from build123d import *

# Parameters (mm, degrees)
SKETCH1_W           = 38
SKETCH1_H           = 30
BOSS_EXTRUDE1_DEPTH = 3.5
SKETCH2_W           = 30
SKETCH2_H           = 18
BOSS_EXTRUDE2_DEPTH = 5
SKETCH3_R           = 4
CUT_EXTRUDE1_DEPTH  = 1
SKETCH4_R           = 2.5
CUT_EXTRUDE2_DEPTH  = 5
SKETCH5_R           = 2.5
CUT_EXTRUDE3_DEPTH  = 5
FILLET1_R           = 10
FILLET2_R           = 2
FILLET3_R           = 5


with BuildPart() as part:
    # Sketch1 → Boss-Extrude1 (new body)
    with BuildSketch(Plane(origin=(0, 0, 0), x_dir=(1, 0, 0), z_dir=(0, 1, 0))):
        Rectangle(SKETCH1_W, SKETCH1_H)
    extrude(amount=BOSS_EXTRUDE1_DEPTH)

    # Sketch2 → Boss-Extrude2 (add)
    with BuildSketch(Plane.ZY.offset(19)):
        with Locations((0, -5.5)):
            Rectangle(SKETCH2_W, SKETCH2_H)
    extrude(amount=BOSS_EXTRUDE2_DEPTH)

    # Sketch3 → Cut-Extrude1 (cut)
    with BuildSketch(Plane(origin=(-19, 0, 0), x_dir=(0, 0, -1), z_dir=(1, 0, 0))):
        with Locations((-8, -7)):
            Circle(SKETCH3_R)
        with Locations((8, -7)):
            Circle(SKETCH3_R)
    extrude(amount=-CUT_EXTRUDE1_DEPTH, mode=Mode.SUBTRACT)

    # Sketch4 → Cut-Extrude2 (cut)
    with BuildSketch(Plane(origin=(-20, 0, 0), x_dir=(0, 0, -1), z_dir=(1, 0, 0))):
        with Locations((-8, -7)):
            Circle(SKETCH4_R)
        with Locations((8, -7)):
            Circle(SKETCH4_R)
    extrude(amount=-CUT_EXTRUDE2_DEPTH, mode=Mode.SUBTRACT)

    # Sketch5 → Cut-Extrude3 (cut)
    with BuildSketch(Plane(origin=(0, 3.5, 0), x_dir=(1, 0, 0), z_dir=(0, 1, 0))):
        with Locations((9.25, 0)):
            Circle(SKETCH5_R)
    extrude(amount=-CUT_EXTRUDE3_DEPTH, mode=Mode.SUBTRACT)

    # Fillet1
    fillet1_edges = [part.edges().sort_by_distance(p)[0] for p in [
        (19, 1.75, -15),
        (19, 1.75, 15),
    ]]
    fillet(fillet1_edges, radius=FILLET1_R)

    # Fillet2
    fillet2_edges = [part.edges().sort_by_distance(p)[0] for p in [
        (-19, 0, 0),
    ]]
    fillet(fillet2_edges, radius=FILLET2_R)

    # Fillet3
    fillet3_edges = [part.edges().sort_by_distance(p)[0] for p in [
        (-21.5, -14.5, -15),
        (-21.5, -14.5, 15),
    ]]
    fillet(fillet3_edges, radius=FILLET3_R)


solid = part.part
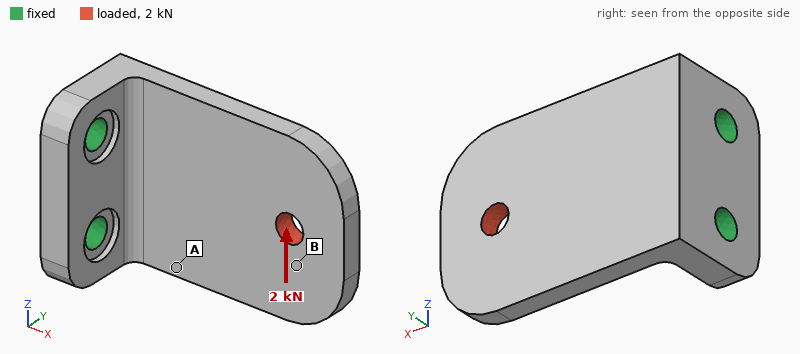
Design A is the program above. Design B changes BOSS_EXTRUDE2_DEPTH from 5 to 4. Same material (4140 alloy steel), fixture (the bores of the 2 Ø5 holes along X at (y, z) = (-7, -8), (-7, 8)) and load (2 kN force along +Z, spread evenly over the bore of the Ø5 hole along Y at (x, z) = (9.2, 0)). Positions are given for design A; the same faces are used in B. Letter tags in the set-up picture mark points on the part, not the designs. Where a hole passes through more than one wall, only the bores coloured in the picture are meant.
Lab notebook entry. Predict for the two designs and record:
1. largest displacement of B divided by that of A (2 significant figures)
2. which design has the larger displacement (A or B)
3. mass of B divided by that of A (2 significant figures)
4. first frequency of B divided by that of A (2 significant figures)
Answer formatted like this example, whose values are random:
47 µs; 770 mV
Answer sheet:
1.4; B; 0.92; 0.90
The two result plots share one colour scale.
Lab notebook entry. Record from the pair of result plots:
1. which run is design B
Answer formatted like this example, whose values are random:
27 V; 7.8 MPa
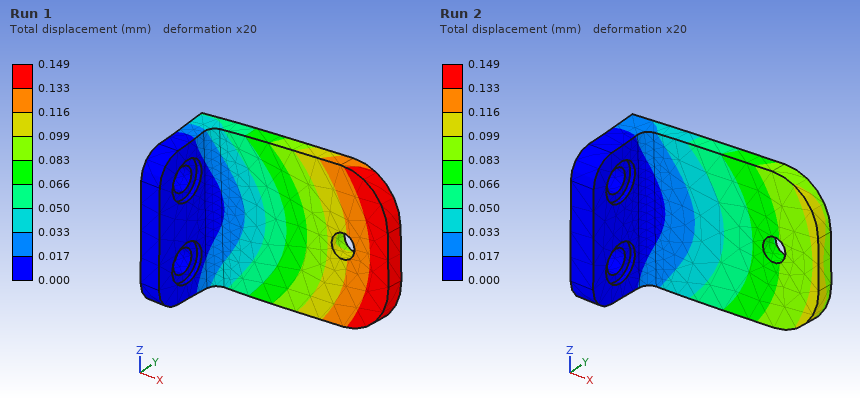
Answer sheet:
Run 1
